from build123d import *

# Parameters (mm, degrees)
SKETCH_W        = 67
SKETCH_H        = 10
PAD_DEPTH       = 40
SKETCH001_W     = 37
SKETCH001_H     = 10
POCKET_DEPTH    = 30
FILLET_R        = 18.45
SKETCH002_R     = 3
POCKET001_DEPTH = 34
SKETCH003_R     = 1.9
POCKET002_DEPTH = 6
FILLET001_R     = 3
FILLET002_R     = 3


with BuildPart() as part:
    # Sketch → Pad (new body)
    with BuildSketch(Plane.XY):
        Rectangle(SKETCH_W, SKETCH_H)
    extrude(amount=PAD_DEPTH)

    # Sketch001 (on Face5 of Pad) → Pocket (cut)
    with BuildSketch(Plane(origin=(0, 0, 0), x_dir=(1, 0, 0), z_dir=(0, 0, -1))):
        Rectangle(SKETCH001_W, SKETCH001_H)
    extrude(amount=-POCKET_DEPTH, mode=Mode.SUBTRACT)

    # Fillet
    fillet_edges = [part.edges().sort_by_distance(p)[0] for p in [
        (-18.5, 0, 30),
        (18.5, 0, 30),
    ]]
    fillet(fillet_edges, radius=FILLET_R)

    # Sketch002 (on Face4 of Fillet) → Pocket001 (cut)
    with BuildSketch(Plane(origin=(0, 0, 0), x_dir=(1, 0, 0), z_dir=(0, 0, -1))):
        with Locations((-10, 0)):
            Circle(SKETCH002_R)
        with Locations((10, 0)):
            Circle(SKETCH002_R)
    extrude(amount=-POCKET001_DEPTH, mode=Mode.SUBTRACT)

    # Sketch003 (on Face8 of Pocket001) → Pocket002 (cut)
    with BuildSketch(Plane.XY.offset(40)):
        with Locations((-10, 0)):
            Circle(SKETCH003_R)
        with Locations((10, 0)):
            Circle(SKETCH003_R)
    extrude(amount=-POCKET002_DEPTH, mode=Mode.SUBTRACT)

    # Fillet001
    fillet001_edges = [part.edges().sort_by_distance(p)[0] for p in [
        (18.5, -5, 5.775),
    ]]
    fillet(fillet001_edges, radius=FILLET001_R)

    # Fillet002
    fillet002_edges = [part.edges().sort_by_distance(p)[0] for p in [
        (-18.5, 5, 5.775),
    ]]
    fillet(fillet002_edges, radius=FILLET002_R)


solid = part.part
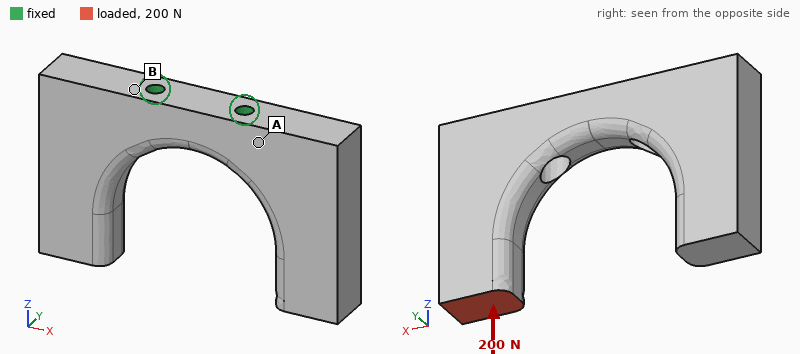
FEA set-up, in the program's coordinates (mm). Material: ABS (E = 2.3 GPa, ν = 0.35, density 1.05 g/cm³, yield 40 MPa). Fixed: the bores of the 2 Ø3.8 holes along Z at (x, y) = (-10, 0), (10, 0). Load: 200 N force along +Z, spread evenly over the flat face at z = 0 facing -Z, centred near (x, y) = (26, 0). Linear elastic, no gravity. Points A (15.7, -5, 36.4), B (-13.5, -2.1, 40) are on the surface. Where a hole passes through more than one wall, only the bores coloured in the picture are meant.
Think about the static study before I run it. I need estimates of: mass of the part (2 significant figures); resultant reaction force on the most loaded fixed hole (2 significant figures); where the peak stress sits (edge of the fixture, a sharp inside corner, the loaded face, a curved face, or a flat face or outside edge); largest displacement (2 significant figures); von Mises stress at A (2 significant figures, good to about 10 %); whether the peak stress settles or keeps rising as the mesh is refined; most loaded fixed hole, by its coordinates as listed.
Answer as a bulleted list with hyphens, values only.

- 17 g
- 290 N
- edge of the fixture
- 0.58 mm
- 5.8 MPa
- keeps rising
- (10, 0)
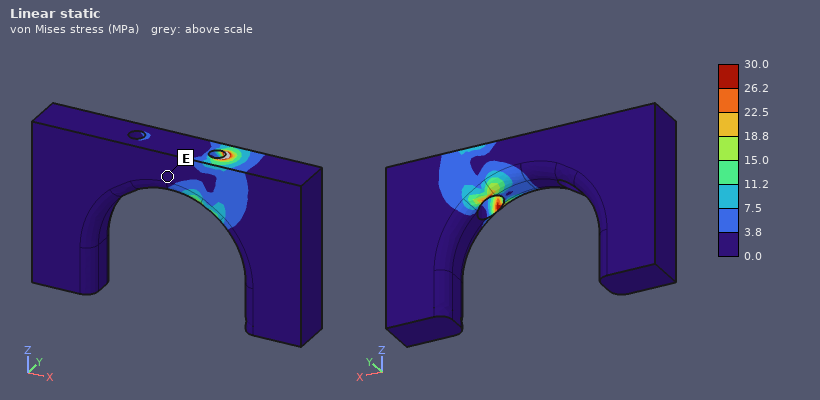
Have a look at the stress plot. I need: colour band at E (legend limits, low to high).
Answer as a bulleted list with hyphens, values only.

- 0.0 to 3.8 MPa
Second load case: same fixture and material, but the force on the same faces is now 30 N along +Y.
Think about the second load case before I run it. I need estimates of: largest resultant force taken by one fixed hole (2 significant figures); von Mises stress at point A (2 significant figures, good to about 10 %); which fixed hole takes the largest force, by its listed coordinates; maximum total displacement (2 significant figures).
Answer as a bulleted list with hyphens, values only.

- 42 N
- 4.9 MPa
- (10, 0)
- 0.44 mm
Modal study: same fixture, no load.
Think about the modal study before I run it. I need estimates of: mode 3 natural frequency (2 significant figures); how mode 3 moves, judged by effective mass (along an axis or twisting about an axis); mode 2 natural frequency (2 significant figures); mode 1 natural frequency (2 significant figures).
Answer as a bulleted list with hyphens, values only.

- 1200 Hz
- along Z
- 990 Hz
- 970 Hz
